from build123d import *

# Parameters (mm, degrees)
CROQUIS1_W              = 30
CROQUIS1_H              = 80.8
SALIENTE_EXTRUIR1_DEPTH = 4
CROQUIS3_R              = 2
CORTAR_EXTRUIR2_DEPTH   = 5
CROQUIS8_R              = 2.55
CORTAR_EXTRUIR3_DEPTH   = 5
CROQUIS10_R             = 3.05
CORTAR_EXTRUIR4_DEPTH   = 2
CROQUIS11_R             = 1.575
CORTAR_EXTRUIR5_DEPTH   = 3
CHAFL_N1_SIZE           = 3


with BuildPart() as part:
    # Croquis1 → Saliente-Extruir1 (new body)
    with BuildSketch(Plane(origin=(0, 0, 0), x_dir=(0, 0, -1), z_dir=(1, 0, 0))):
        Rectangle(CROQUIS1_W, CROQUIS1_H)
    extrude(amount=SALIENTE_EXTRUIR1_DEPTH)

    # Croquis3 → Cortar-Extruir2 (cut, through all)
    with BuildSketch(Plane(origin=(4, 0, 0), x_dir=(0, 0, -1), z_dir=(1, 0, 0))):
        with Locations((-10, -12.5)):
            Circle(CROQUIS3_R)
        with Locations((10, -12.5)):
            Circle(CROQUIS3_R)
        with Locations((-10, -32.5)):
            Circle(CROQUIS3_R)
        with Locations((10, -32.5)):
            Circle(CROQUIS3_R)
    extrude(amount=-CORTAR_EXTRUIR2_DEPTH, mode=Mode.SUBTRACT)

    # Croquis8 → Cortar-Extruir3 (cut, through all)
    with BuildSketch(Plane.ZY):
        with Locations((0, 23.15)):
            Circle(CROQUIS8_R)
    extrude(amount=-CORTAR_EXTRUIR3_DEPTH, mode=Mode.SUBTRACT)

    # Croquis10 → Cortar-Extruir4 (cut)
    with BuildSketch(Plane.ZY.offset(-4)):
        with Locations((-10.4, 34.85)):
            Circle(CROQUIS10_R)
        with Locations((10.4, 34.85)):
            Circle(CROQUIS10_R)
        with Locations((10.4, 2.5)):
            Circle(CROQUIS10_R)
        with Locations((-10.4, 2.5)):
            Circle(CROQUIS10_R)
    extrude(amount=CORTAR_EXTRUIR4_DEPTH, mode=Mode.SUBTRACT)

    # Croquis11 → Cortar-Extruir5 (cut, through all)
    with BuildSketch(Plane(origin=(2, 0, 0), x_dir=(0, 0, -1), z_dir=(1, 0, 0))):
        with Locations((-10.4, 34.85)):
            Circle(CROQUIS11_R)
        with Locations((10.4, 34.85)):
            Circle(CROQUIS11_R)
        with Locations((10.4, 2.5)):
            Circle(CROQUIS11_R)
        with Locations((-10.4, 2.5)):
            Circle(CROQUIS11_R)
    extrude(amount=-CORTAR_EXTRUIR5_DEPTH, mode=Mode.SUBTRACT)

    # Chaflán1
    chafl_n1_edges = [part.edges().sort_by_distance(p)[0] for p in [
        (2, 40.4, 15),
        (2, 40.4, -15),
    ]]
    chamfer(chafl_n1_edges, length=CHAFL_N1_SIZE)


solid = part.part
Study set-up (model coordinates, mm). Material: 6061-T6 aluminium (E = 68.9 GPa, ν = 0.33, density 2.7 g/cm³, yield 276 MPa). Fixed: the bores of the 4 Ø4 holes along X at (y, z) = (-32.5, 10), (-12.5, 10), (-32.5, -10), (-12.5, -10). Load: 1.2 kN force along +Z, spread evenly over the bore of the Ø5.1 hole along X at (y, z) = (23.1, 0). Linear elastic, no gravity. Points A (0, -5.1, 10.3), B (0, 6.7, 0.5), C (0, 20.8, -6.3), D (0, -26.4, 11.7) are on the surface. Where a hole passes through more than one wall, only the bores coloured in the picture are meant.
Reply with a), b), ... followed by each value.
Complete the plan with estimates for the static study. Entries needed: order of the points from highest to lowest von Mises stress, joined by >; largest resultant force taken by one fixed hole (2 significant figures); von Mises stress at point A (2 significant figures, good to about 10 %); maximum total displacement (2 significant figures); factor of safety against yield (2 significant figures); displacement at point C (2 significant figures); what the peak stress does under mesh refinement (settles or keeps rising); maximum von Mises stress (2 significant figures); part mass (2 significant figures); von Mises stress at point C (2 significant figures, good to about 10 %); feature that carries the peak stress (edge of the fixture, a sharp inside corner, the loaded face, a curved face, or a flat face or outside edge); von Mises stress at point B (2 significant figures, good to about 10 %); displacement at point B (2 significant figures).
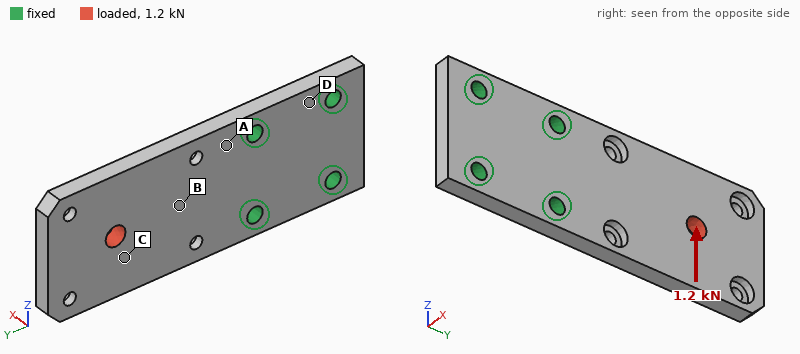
a) A > B > C > D
b) 1.9 kN
c) 45 MPa
d) 80 µm
e) 1.9
f) 48 µm
g) settles
h) 140 MPa
i) 25 g
j) 21 MPa
k) a curved face
l) 33 MPa
m) 20 µm
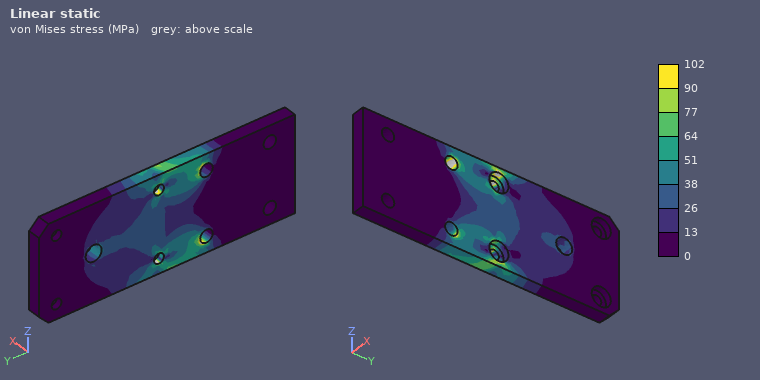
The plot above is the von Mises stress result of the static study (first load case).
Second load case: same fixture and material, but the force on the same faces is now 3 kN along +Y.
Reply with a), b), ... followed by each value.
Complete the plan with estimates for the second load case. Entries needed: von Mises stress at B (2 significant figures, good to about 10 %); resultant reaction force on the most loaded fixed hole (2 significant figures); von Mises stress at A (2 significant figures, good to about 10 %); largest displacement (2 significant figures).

a) 28 MPa
b) 1.4 kN
c) 26 MPa
d) 29 µm
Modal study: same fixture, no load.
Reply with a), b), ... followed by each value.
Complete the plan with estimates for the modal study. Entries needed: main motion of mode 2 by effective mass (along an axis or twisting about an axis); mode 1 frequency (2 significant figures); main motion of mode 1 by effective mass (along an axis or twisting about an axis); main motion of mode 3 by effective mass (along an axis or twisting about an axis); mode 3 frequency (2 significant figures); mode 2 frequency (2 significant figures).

a) twisting about Y
b) 1200 Hz
c) along X
d) along Z
e) 7000 Hz
f) 4400 Hz
